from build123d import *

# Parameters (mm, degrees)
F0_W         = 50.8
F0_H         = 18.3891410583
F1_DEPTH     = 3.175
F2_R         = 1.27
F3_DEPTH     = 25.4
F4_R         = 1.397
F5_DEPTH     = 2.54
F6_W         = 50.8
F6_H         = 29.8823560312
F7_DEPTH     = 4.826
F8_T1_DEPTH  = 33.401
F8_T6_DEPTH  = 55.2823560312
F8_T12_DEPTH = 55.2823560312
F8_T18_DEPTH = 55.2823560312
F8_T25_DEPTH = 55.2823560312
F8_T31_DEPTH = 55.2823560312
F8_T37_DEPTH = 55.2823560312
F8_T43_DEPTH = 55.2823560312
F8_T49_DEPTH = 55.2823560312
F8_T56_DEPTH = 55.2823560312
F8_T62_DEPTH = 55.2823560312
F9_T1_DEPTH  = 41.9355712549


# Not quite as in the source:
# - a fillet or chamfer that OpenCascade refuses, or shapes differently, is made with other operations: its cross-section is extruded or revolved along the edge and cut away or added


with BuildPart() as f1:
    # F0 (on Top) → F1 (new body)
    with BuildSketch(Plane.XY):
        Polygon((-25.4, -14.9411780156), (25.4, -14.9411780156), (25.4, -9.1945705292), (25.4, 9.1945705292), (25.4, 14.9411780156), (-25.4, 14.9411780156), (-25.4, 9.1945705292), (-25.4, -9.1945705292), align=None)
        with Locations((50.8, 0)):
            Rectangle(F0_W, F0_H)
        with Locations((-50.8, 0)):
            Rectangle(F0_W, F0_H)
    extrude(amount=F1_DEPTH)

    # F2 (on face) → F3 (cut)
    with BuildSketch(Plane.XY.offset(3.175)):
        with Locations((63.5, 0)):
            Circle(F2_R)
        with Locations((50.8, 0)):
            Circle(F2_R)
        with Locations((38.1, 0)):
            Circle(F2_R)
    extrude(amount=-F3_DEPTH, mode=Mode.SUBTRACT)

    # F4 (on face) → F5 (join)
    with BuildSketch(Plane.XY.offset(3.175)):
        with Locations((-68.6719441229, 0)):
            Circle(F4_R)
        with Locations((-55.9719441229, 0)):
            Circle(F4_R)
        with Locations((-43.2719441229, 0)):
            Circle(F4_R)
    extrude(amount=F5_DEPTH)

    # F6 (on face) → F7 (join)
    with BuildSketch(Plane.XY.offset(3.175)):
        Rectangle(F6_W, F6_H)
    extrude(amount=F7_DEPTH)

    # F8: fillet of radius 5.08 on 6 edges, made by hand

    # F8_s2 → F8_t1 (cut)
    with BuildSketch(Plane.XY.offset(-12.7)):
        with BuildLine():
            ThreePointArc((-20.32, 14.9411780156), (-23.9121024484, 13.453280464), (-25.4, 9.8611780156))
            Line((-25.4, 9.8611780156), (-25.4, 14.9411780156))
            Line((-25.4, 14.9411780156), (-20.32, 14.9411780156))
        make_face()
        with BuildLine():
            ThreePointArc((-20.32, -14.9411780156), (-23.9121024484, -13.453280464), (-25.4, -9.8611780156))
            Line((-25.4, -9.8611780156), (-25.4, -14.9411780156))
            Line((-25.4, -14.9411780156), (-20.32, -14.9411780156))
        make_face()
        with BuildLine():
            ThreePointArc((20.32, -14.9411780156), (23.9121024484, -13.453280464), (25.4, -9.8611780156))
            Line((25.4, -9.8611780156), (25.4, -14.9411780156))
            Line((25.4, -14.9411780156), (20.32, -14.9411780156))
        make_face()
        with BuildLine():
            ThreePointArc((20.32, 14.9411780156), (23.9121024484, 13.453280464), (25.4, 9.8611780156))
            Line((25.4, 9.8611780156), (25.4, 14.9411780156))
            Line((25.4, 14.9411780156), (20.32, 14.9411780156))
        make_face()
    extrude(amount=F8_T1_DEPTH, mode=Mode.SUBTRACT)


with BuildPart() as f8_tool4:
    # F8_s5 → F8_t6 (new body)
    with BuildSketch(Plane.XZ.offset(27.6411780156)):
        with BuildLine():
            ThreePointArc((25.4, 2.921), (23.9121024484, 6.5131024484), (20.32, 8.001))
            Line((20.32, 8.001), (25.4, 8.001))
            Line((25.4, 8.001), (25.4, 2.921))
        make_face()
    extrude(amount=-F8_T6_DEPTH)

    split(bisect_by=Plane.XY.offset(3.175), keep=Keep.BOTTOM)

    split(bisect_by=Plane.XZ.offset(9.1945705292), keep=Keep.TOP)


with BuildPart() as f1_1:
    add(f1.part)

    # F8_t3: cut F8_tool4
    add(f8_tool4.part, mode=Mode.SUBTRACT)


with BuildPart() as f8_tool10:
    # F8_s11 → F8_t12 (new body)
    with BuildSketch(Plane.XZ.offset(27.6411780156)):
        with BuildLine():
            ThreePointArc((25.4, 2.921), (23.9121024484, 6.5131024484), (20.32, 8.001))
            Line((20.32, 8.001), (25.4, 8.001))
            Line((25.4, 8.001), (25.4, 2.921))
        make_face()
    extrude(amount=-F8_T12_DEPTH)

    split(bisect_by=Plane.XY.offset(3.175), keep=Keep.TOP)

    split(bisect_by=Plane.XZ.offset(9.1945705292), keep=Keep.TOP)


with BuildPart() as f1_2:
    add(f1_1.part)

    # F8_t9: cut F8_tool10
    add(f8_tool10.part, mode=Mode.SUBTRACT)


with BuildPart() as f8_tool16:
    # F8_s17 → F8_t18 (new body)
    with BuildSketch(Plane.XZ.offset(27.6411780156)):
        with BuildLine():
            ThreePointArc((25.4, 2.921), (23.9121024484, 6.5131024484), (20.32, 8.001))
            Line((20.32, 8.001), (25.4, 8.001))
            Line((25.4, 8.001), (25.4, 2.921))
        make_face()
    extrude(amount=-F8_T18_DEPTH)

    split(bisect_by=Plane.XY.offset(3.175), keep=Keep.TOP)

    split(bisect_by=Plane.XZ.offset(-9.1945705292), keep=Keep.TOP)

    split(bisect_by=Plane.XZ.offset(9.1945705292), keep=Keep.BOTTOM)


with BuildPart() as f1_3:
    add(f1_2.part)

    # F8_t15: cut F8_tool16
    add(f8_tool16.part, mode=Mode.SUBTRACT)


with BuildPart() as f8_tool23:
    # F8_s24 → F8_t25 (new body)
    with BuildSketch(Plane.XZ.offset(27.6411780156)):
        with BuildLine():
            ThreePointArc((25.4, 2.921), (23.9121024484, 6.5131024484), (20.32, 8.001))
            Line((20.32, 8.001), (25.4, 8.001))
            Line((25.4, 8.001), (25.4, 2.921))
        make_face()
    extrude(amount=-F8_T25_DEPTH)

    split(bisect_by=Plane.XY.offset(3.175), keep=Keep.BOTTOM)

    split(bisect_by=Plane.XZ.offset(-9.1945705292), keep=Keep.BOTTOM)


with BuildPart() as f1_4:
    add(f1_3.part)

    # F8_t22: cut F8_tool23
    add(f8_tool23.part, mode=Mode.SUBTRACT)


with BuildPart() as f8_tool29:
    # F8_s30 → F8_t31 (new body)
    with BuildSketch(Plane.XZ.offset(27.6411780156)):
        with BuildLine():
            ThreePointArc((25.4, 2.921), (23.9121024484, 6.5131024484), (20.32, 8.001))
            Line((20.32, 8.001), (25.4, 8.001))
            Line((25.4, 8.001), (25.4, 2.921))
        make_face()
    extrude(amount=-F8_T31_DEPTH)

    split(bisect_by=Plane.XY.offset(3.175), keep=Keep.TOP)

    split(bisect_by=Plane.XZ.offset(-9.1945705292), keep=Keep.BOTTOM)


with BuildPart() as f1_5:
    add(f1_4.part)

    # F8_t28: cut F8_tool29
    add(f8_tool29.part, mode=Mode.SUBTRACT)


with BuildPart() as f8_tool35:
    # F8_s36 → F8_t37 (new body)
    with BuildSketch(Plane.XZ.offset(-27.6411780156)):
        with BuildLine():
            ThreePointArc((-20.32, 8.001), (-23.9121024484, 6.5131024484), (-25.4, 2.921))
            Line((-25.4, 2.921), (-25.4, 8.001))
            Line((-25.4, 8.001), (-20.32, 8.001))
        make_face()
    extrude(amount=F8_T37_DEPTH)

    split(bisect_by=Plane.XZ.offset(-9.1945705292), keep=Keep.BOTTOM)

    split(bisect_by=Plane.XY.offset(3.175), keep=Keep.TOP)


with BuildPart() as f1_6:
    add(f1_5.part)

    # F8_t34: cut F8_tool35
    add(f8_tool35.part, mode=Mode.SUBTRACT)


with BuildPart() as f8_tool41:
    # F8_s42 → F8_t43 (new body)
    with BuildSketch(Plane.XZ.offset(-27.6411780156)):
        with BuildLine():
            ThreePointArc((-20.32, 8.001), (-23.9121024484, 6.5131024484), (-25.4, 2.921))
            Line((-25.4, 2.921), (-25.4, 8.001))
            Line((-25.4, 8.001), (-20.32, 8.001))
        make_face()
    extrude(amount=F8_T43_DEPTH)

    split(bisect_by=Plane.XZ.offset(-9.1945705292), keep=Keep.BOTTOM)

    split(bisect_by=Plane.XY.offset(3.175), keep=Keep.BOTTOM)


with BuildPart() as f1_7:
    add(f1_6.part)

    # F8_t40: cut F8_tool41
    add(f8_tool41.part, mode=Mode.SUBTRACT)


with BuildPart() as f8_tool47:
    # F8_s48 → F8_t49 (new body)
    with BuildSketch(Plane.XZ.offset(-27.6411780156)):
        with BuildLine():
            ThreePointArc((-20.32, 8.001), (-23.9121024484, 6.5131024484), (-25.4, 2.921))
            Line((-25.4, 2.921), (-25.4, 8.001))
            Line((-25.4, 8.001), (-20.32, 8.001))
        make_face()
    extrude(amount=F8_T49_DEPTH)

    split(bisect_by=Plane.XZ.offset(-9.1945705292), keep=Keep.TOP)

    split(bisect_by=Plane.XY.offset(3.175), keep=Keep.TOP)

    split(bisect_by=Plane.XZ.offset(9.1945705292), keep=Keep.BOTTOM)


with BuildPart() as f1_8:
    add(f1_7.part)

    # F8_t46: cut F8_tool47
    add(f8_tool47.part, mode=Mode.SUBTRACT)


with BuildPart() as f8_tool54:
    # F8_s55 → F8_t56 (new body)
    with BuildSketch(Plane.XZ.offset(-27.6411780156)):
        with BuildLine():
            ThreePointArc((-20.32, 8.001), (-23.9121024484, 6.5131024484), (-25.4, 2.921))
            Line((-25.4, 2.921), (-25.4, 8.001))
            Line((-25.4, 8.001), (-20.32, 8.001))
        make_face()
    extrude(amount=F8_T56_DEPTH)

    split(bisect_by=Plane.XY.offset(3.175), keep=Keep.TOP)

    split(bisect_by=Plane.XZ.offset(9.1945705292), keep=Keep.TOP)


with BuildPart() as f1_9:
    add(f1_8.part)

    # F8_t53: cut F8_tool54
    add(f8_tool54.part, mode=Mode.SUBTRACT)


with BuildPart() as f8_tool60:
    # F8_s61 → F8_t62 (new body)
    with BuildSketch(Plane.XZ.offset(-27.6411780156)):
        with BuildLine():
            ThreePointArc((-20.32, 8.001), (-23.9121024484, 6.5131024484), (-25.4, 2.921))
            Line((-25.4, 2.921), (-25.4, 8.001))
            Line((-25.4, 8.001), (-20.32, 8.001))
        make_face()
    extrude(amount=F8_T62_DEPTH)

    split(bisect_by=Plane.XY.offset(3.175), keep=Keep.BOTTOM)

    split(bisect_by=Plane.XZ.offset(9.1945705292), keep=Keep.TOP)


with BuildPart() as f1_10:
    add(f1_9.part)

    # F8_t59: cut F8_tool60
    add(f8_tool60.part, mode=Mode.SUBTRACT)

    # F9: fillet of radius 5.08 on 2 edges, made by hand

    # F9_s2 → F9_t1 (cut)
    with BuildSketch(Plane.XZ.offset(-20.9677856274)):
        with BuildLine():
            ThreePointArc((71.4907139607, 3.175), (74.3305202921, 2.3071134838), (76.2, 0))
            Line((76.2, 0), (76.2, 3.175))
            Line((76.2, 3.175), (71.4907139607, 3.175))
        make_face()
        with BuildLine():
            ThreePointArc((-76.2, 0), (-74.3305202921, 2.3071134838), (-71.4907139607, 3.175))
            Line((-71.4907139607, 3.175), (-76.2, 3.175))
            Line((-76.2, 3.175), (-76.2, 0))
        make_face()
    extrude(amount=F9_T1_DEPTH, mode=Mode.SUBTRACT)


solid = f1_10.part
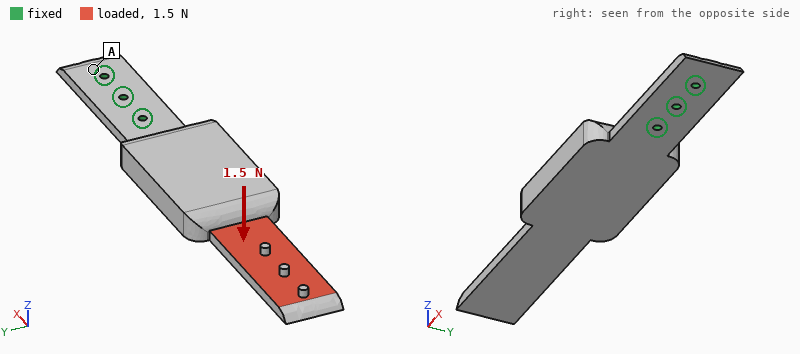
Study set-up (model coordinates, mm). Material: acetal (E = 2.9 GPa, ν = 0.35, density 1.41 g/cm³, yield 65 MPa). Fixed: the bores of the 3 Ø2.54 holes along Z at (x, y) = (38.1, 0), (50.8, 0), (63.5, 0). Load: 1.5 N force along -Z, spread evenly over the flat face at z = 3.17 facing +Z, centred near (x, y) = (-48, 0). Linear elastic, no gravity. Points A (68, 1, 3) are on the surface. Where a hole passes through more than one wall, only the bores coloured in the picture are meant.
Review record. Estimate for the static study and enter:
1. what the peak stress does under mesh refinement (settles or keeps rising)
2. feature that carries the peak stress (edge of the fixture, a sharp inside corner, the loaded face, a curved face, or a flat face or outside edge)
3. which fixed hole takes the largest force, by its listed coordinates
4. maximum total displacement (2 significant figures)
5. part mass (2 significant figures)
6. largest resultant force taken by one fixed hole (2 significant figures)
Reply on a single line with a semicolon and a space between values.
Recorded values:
keeps rising; edge of the fixture; (38.1, 0); 1.5 mm; 25 g; 5.8 N
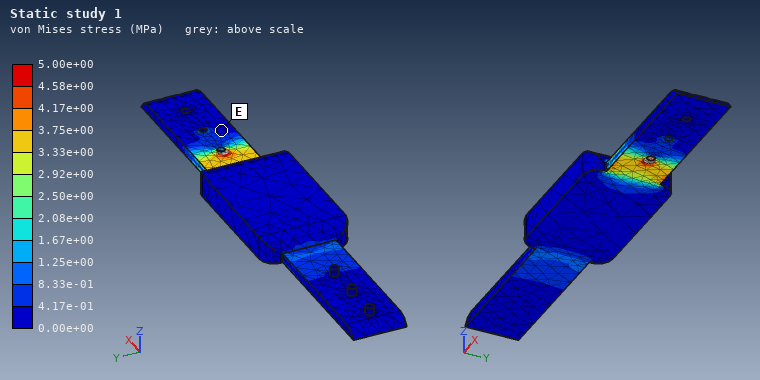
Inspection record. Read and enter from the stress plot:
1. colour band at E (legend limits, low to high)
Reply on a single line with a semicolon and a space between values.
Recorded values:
0.00e+00 to 4.17e-01 MPa
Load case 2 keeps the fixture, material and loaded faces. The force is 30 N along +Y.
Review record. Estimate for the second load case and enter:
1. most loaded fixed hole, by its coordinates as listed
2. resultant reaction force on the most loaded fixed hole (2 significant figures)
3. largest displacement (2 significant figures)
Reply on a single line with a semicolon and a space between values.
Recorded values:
(38.1, 0); 160 N; 1.7 mm
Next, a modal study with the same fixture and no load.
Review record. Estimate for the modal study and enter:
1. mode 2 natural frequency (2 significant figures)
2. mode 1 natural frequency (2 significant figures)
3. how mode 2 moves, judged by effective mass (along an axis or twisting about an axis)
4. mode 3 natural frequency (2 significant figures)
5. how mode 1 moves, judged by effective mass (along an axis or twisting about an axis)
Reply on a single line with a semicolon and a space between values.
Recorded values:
280 Hz; 70 Hz; along Y; 370 Hz; along Z
